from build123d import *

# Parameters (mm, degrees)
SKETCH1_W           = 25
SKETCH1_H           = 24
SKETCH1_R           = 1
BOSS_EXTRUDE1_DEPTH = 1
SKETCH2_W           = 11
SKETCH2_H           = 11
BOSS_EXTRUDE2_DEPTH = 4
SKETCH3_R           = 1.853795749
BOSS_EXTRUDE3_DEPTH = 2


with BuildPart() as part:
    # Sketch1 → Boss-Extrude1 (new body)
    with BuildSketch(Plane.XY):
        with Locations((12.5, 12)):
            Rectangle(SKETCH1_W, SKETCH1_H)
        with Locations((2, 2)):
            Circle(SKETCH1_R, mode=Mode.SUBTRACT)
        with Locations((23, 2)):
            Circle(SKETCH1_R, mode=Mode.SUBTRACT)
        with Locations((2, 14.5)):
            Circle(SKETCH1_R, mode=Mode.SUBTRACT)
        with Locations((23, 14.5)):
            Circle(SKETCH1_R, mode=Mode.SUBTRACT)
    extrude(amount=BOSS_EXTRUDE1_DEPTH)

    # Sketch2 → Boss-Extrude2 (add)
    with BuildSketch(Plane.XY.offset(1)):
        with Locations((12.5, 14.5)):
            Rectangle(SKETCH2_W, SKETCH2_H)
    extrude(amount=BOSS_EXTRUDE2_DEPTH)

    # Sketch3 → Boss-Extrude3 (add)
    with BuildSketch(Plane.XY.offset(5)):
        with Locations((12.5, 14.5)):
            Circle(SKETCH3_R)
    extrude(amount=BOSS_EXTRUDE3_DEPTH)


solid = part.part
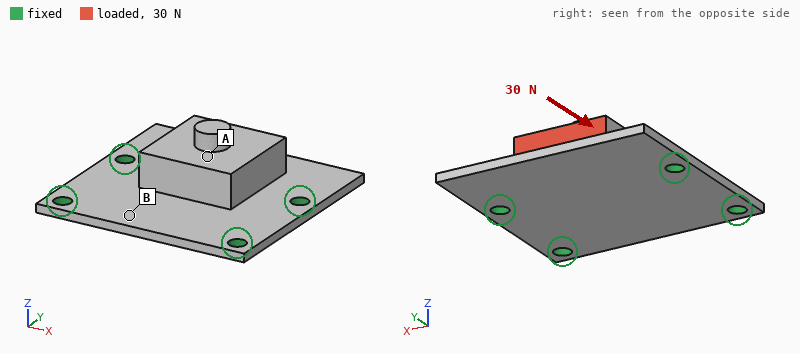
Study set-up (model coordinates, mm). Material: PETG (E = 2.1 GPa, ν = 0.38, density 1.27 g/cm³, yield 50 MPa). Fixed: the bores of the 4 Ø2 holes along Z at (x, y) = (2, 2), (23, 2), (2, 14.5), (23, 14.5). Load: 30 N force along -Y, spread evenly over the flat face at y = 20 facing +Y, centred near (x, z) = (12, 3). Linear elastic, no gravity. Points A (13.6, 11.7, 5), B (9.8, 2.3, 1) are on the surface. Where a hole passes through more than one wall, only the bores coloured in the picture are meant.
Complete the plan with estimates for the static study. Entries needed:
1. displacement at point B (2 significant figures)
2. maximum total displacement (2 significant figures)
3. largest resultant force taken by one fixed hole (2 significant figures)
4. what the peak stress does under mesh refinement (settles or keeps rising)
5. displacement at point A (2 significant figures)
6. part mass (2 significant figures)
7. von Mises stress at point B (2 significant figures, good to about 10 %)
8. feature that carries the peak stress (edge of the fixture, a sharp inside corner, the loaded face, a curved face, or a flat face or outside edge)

0.058 mm
0.17 mm
9.7 N
keeps rising
0.077 mm
1.4 g
2.0 MPa
edge of the fixture
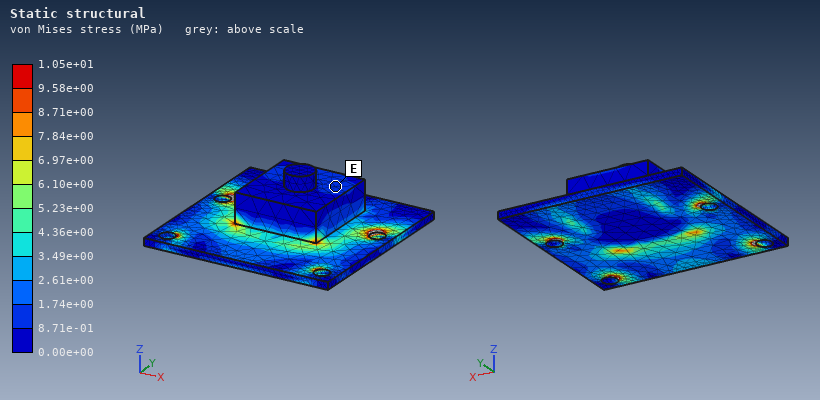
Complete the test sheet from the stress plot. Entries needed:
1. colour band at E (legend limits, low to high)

8.71e-01 to 1.74e+00 MPa
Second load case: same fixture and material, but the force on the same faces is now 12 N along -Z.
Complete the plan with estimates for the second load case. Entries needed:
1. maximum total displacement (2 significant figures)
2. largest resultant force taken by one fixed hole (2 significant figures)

0.23 mm
9.2 N
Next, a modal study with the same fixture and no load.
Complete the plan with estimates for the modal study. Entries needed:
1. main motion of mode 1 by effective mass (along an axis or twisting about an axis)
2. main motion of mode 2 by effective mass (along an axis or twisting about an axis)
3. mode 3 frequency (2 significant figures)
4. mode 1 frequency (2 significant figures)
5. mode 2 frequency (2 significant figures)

along Z
along Z
4300 Hz
2100 Hz
2900 Hz
